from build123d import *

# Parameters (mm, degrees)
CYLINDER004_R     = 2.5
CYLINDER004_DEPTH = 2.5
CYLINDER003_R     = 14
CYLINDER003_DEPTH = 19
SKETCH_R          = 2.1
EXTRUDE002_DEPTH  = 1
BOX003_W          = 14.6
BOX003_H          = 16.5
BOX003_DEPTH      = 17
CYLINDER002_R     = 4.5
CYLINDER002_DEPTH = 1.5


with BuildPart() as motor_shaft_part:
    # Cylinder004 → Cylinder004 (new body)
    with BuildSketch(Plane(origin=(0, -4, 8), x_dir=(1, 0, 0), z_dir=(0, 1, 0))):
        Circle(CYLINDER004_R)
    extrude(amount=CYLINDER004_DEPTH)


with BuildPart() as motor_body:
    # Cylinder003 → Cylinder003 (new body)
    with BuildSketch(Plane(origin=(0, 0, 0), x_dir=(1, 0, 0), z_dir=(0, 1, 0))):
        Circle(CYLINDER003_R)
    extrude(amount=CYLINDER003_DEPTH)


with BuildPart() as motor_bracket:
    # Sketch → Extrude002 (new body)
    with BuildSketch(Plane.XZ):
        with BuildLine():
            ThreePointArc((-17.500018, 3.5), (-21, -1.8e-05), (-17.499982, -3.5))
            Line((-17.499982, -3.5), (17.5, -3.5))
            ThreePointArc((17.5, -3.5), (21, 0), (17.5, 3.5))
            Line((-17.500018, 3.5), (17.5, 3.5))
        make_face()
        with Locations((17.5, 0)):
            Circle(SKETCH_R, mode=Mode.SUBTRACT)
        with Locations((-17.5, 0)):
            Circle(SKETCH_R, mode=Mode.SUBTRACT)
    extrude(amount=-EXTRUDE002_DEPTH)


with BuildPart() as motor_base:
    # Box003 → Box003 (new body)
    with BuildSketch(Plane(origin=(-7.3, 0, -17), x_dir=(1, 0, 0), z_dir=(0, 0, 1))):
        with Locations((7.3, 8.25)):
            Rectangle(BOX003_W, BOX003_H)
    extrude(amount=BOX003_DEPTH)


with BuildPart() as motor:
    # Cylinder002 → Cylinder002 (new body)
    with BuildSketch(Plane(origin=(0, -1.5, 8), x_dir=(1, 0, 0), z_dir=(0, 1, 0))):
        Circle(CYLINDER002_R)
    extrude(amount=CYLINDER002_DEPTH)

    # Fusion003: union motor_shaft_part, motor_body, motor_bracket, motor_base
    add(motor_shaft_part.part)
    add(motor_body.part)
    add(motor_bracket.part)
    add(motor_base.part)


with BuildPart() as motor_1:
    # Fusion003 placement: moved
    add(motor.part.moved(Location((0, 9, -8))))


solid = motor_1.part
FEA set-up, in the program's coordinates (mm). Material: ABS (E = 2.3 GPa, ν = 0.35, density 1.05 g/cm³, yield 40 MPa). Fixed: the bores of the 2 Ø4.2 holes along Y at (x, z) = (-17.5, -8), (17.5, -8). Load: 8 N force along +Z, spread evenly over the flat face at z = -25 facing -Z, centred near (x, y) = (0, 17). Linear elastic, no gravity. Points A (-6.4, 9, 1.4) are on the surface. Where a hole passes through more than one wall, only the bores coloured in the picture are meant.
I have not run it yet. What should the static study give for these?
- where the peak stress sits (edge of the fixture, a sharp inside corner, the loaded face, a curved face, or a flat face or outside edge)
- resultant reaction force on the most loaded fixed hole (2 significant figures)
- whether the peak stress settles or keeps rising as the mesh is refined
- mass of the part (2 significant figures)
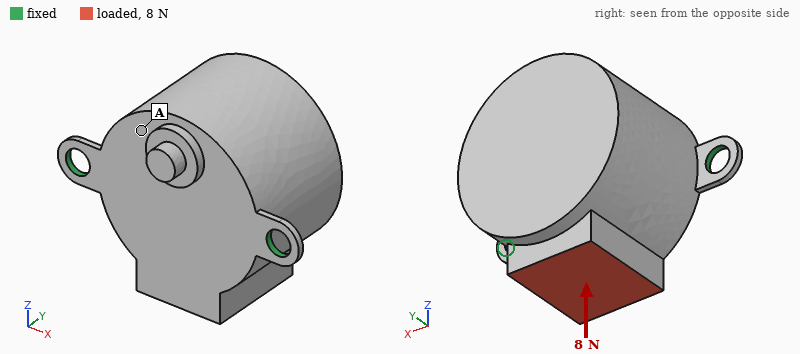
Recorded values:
edge of the fixture
4.0 N
keeps rising
13 g
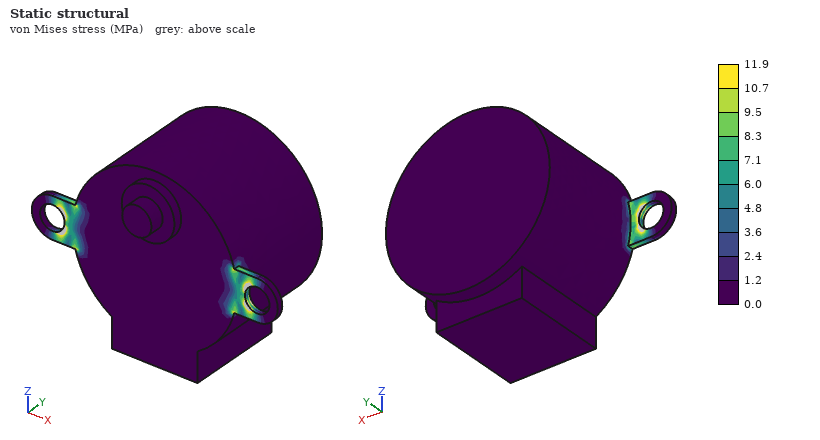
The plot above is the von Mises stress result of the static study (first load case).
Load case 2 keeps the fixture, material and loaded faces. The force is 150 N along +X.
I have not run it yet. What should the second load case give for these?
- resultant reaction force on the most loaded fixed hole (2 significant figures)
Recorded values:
120 N
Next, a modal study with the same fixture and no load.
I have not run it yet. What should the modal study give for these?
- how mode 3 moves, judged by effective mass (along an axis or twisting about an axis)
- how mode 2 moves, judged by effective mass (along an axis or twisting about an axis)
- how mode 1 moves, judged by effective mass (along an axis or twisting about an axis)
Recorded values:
along X
along Y
along Z
